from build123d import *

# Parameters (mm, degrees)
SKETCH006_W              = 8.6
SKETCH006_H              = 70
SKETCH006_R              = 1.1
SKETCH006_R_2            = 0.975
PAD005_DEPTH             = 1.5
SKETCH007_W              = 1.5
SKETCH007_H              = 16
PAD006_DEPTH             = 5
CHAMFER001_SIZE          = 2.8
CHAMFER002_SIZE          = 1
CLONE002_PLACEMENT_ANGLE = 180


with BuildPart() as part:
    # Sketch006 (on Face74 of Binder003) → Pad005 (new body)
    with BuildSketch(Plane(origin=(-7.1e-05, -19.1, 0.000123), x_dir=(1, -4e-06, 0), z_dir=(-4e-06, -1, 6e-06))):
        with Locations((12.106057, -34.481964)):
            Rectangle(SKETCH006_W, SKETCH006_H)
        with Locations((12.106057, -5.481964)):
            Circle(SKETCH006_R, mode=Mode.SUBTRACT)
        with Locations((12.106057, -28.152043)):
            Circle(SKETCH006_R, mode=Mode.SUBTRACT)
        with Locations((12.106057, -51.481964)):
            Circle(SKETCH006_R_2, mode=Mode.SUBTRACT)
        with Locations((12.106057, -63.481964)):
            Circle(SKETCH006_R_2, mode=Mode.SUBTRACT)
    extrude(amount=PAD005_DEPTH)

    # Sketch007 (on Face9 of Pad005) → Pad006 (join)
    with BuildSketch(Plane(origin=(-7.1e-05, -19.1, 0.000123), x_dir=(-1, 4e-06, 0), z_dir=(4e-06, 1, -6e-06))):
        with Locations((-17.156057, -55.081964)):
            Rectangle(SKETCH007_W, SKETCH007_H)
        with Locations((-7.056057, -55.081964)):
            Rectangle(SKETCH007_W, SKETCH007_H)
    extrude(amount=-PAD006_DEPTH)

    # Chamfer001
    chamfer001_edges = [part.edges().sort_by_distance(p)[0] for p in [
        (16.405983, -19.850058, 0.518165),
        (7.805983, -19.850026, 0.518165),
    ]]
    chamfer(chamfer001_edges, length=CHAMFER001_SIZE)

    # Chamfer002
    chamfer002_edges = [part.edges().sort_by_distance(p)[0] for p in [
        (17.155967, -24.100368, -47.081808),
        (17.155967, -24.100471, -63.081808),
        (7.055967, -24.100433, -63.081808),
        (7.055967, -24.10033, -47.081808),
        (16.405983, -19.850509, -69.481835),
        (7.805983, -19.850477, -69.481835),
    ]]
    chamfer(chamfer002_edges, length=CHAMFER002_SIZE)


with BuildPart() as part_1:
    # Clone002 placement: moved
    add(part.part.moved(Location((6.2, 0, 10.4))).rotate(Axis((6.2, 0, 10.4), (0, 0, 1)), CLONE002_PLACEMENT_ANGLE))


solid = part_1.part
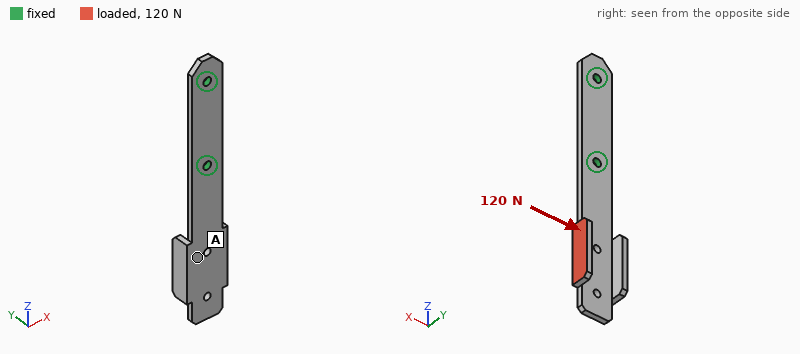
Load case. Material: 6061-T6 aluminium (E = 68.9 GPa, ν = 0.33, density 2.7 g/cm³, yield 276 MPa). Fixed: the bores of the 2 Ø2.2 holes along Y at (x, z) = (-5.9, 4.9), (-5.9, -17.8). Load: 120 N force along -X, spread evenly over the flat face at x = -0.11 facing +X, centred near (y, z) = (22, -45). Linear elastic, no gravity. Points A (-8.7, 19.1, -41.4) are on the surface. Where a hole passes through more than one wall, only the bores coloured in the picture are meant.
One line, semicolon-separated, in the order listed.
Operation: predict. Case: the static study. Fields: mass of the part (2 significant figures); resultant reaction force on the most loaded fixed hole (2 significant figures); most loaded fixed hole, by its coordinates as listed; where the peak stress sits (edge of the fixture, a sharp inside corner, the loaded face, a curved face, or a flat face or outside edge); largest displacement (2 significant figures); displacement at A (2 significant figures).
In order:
3.0 g; 200 N; (-5.9, -17.8); edge of the fixture; 0.40 mm; 0.18 mm
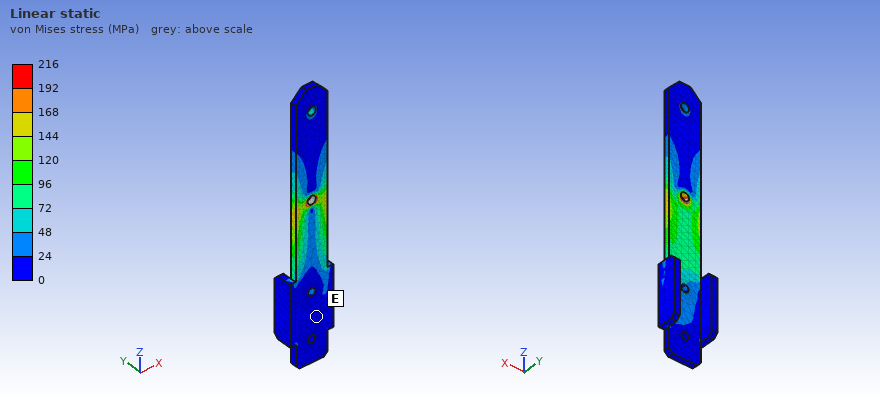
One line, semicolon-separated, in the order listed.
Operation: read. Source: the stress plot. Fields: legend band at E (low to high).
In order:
0 to 24 MPa
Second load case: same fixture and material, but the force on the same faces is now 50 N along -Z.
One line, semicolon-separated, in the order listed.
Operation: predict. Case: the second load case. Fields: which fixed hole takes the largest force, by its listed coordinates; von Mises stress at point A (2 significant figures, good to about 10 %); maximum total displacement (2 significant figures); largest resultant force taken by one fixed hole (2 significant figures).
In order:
(-5.9, -17.8); 7.3 MPa; 0.33 mm; 48 N
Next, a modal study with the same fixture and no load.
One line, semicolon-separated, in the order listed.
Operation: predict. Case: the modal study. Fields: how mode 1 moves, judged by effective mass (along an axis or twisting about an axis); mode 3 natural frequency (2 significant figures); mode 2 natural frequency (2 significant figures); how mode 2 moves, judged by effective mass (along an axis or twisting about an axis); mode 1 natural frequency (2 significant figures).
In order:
along Y; 3400 Hz; 2700 Hz; along X; 610 Hz
